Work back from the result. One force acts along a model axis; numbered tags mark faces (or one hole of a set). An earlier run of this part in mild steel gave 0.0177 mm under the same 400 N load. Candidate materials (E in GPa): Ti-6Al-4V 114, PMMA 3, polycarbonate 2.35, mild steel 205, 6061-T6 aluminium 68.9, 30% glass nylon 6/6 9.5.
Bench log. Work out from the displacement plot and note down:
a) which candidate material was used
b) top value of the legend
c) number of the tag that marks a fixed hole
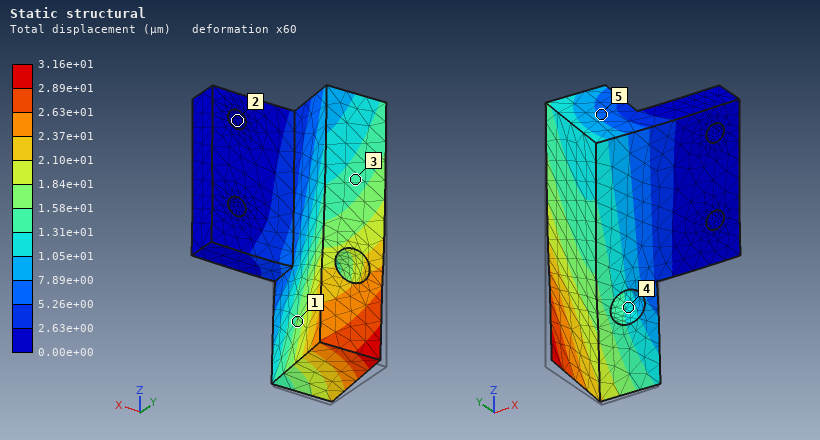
Ti-6Al-4V
3.16e+01 µm
2
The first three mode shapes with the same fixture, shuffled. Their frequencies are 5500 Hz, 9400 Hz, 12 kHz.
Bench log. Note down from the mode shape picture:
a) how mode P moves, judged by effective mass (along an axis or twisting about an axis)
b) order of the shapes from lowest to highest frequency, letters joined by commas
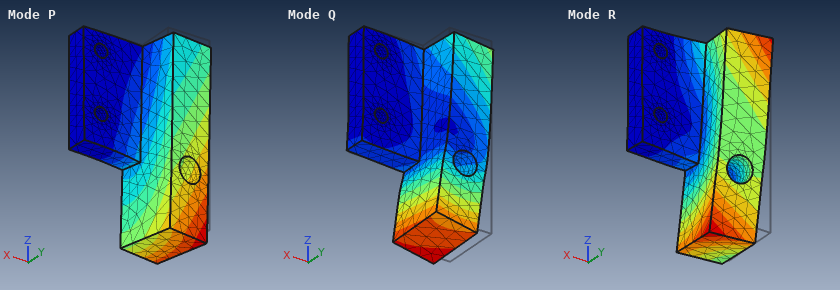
along Y
P, R, Q
